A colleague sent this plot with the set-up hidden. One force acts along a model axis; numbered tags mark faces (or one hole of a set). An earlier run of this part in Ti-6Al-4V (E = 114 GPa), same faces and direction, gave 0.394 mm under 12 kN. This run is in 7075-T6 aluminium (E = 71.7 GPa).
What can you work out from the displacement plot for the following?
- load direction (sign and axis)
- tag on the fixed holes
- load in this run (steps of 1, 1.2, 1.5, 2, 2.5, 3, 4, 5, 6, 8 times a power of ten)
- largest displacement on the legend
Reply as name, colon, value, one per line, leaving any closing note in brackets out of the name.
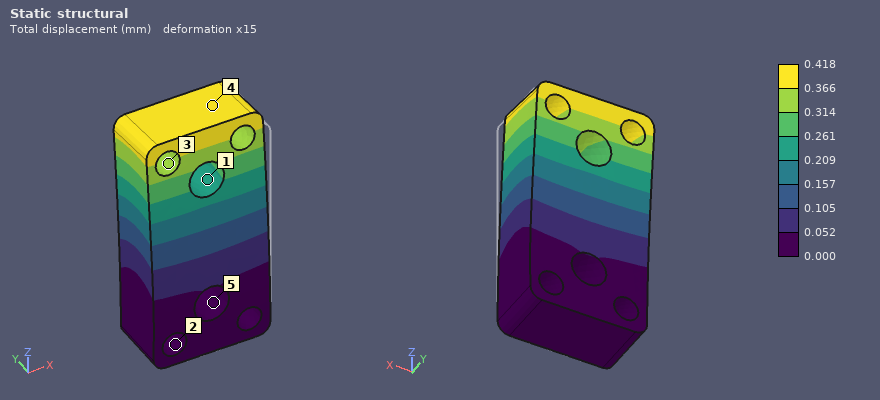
load direction: +Y
tag on the fixed holes: 2
load in this run: 8 kN
largest displacement on the legend: 0.418 mm
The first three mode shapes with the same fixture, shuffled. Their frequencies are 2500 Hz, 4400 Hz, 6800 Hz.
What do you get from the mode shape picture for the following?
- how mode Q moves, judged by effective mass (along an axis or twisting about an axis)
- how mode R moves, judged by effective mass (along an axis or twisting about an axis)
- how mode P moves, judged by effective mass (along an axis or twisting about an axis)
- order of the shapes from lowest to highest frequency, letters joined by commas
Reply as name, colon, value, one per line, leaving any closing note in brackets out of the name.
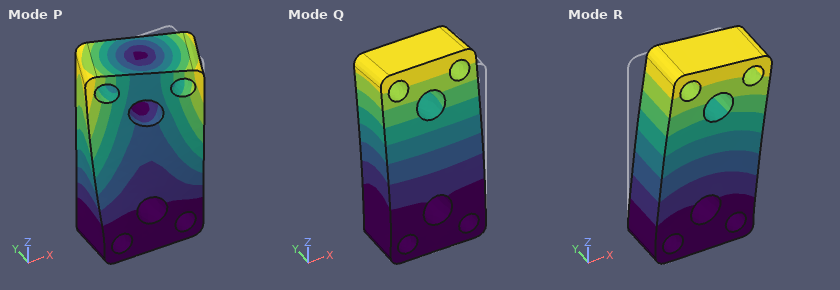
how mode Q moves, judged by effective mass: along Y
how mode R moves, judged by effective mass: along X
how mode P moves, judged by effective mass: twisting about Z
order of the shapes from lowest to highest frequency, letters joined by commas: Q, R, P
